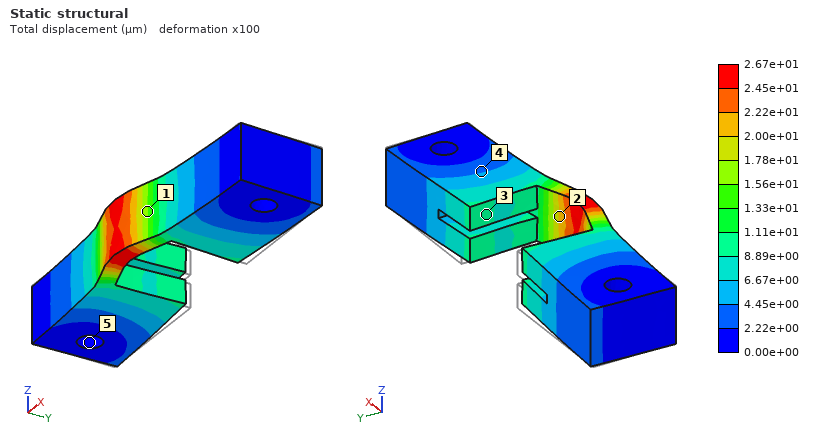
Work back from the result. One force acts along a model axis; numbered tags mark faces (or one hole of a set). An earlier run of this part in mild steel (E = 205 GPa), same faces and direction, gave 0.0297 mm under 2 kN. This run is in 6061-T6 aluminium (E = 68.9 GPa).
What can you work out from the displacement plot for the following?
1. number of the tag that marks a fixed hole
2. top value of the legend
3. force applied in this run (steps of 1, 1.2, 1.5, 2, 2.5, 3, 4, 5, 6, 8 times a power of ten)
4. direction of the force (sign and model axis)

5
2.67e+01 µm
600 N
-Y
